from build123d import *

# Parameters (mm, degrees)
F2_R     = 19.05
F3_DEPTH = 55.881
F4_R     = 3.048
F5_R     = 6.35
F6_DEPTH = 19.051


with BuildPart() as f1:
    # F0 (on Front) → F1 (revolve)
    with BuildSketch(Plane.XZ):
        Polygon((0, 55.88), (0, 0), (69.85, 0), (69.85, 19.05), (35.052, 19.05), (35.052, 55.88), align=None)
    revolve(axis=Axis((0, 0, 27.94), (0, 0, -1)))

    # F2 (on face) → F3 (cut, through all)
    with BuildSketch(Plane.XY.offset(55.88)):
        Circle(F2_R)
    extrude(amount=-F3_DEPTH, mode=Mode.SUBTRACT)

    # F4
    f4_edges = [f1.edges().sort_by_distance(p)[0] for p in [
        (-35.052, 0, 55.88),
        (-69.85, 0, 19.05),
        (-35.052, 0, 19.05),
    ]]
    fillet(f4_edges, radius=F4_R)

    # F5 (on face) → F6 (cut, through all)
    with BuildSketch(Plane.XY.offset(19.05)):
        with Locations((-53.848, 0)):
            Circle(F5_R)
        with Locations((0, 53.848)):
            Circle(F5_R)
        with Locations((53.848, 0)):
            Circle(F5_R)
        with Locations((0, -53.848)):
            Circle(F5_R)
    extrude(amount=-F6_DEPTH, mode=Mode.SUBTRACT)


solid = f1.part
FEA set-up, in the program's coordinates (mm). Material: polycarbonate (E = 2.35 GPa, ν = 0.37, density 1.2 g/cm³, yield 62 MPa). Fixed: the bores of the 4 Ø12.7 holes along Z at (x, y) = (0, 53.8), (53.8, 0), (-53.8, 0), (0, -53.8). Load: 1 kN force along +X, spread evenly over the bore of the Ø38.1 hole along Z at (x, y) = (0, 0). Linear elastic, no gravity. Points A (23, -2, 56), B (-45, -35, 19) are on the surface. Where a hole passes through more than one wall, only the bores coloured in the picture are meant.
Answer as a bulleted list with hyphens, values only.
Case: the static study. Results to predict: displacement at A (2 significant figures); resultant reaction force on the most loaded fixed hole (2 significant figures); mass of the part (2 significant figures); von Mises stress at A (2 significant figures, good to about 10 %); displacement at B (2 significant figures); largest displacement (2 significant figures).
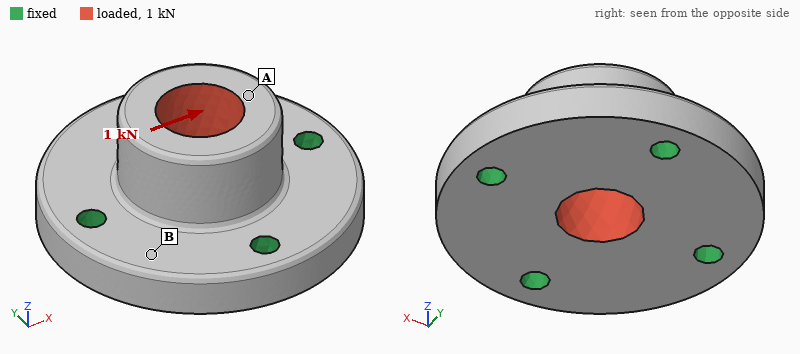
- 26 µm
- 370 N
- 430 g
- 0.38 MPa
- 5.7 µm
- 26 µm
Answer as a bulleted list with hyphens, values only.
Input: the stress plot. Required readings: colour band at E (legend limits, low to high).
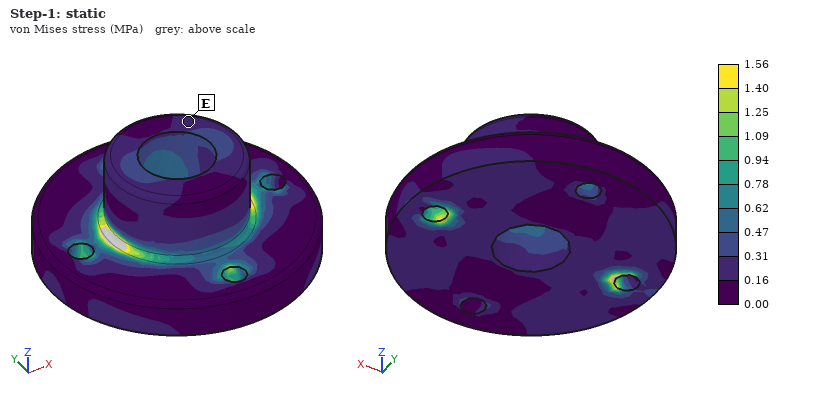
- 0.16 to 0.31 MPa
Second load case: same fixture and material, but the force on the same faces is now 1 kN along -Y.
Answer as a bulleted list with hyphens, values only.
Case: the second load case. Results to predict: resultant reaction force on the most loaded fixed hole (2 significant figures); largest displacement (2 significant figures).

- 370 N
- 26 µm
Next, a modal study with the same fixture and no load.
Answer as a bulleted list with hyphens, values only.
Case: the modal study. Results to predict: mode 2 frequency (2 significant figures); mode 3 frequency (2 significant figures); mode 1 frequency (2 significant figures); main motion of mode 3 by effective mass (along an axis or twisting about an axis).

- 2500 Hz
- 2600 Hz
- 2500 Hz
- along Z
